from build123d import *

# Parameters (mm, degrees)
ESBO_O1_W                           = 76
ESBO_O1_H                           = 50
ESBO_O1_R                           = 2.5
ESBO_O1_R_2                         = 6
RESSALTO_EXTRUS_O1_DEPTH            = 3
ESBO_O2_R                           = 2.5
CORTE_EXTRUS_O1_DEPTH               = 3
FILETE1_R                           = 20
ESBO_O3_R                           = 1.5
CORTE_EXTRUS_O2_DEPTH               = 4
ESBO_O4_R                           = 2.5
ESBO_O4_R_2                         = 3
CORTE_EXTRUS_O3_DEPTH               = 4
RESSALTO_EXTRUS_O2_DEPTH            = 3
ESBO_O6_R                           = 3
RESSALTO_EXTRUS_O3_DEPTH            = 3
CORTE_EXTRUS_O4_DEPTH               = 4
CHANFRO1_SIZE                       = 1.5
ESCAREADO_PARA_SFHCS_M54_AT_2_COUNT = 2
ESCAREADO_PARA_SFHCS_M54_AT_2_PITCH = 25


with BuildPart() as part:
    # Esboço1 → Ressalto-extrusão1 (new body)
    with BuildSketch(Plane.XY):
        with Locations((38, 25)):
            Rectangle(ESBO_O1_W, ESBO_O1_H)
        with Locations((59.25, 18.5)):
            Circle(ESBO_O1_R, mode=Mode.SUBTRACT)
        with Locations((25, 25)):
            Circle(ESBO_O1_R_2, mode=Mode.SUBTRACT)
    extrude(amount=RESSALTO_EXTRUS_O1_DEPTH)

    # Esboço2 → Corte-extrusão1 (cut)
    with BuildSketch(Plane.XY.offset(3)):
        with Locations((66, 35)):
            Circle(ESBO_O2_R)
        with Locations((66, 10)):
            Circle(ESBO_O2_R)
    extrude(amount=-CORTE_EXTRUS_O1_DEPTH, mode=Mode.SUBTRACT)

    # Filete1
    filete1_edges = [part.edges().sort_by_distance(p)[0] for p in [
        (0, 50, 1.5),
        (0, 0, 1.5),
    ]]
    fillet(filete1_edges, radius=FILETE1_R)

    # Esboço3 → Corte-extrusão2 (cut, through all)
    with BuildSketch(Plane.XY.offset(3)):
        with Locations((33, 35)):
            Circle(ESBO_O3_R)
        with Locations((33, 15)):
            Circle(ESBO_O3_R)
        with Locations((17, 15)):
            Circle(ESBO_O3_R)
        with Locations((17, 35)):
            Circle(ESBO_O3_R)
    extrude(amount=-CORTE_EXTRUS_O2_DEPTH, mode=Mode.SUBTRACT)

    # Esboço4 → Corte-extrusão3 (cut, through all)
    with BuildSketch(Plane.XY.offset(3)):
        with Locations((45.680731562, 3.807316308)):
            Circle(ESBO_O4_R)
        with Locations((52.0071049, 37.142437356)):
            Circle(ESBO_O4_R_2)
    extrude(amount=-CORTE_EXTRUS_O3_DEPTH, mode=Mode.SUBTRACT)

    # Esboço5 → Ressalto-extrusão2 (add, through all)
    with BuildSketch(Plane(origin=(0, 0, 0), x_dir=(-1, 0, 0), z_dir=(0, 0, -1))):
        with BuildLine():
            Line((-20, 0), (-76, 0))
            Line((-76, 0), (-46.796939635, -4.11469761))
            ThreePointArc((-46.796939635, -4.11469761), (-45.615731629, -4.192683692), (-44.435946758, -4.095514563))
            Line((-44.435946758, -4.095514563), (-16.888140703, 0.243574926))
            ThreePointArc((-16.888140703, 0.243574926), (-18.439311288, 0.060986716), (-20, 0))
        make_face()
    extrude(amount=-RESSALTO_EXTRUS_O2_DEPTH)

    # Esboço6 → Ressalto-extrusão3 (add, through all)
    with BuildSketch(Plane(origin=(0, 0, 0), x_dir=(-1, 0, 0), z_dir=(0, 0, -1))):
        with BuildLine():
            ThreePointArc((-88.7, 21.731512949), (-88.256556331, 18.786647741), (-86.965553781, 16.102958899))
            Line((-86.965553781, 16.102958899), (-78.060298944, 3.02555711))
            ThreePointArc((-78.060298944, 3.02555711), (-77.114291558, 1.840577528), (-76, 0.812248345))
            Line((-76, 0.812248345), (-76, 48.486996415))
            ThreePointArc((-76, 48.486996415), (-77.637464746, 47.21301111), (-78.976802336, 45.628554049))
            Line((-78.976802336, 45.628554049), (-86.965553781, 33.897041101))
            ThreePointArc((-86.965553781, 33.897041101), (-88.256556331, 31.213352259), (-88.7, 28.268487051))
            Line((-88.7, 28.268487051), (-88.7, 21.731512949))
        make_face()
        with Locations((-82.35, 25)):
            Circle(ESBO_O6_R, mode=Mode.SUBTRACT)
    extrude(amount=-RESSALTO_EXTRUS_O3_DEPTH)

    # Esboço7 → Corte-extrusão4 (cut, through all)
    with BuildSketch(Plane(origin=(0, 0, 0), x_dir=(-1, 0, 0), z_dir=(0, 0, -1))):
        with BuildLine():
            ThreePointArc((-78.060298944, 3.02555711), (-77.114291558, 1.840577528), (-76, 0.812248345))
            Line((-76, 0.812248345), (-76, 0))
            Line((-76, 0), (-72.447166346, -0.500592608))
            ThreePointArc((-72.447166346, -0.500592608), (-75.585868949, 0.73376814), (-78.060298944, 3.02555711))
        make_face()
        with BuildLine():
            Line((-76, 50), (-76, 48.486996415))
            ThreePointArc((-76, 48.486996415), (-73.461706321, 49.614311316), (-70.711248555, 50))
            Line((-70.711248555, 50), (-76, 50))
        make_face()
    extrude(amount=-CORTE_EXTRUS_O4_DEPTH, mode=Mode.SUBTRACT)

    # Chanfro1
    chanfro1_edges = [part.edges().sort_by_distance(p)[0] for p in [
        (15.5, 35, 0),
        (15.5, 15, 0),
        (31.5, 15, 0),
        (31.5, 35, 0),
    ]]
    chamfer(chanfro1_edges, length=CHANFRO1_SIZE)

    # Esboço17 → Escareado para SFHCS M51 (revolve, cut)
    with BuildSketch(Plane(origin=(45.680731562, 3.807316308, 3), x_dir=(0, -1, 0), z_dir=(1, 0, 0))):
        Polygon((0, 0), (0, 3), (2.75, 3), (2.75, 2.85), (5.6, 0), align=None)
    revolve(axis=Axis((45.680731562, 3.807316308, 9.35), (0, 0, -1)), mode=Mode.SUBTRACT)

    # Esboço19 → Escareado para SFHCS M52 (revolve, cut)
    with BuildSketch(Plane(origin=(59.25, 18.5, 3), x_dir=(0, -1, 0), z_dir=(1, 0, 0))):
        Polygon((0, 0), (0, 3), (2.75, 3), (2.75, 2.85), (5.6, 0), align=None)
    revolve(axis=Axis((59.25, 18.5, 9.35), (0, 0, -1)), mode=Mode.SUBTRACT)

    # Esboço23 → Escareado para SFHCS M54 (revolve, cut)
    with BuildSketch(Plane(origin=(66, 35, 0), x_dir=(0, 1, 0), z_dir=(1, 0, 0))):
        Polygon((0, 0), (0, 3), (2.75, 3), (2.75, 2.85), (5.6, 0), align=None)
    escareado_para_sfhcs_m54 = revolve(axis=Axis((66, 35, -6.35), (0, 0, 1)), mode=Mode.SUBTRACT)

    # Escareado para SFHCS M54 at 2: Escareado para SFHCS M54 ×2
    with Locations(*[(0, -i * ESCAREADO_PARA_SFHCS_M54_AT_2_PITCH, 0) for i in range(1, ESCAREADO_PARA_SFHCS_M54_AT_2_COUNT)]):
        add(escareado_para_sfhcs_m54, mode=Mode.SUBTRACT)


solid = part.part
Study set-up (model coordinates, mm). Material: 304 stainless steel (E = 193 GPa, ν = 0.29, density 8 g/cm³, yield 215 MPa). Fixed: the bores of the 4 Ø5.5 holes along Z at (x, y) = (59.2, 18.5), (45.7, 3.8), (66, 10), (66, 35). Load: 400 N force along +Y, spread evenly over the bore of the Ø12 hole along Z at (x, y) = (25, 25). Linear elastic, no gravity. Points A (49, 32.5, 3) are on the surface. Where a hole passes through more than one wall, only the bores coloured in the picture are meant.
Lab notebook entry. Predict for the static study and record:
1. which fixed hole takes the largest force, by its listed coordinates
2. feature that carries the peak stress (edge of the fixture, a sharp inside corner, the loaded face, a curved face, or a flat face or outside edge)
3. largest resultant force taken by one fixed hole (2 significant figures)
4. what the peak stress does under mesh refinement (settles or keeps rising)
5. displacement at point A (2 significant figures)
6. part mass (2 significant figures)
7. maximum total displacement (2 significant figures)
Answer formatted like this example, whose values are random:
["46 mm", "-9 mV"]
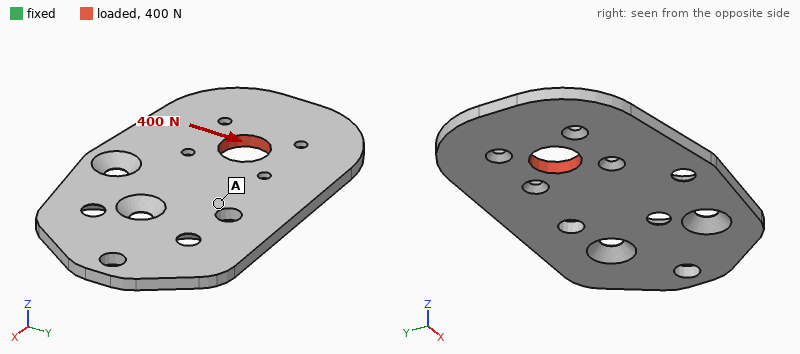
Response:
["(45.7, 3.8)", "edge of the fixture", "390 N", "keeps rising", "4.8 µm", "89 g", "24 µm"]
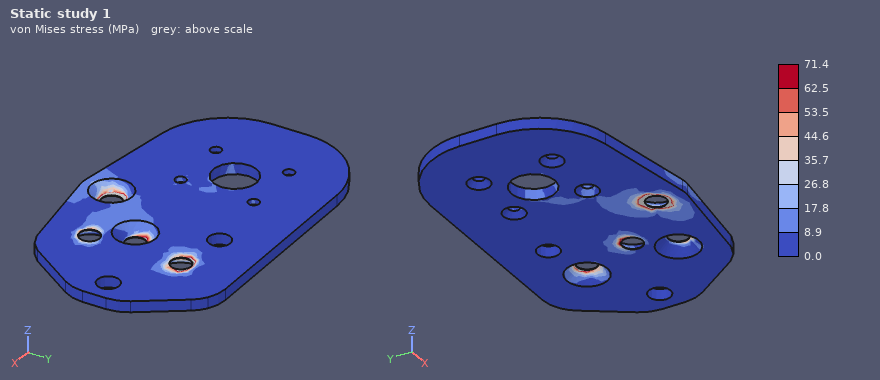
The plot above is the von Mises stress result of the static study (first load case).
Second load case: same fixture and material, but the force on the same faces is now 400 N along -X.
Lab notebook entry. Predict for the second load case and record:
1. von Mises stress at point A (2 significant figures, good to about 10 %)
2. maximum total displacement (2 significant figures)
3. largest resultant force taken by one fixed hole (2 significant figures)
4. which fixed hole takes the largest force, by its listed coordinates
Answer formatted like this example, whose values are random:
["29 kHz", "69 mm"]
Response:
["4.7 MPa", "2.3 µm", "170 N", "(66, 35)"]
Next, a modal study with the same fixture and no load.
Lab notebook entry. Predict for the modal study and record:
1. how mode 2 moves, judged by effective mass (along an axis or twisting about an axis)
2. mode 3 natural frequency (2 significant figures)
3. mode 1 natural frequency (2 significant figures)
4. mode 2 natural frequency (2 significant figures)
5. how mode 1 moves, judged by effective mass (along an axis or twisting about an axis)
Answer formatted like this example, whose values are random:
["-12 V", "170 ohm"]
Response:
["twisting about X", "3900 Hz", "740 Hz", "2100 Hz", "along Z"]
